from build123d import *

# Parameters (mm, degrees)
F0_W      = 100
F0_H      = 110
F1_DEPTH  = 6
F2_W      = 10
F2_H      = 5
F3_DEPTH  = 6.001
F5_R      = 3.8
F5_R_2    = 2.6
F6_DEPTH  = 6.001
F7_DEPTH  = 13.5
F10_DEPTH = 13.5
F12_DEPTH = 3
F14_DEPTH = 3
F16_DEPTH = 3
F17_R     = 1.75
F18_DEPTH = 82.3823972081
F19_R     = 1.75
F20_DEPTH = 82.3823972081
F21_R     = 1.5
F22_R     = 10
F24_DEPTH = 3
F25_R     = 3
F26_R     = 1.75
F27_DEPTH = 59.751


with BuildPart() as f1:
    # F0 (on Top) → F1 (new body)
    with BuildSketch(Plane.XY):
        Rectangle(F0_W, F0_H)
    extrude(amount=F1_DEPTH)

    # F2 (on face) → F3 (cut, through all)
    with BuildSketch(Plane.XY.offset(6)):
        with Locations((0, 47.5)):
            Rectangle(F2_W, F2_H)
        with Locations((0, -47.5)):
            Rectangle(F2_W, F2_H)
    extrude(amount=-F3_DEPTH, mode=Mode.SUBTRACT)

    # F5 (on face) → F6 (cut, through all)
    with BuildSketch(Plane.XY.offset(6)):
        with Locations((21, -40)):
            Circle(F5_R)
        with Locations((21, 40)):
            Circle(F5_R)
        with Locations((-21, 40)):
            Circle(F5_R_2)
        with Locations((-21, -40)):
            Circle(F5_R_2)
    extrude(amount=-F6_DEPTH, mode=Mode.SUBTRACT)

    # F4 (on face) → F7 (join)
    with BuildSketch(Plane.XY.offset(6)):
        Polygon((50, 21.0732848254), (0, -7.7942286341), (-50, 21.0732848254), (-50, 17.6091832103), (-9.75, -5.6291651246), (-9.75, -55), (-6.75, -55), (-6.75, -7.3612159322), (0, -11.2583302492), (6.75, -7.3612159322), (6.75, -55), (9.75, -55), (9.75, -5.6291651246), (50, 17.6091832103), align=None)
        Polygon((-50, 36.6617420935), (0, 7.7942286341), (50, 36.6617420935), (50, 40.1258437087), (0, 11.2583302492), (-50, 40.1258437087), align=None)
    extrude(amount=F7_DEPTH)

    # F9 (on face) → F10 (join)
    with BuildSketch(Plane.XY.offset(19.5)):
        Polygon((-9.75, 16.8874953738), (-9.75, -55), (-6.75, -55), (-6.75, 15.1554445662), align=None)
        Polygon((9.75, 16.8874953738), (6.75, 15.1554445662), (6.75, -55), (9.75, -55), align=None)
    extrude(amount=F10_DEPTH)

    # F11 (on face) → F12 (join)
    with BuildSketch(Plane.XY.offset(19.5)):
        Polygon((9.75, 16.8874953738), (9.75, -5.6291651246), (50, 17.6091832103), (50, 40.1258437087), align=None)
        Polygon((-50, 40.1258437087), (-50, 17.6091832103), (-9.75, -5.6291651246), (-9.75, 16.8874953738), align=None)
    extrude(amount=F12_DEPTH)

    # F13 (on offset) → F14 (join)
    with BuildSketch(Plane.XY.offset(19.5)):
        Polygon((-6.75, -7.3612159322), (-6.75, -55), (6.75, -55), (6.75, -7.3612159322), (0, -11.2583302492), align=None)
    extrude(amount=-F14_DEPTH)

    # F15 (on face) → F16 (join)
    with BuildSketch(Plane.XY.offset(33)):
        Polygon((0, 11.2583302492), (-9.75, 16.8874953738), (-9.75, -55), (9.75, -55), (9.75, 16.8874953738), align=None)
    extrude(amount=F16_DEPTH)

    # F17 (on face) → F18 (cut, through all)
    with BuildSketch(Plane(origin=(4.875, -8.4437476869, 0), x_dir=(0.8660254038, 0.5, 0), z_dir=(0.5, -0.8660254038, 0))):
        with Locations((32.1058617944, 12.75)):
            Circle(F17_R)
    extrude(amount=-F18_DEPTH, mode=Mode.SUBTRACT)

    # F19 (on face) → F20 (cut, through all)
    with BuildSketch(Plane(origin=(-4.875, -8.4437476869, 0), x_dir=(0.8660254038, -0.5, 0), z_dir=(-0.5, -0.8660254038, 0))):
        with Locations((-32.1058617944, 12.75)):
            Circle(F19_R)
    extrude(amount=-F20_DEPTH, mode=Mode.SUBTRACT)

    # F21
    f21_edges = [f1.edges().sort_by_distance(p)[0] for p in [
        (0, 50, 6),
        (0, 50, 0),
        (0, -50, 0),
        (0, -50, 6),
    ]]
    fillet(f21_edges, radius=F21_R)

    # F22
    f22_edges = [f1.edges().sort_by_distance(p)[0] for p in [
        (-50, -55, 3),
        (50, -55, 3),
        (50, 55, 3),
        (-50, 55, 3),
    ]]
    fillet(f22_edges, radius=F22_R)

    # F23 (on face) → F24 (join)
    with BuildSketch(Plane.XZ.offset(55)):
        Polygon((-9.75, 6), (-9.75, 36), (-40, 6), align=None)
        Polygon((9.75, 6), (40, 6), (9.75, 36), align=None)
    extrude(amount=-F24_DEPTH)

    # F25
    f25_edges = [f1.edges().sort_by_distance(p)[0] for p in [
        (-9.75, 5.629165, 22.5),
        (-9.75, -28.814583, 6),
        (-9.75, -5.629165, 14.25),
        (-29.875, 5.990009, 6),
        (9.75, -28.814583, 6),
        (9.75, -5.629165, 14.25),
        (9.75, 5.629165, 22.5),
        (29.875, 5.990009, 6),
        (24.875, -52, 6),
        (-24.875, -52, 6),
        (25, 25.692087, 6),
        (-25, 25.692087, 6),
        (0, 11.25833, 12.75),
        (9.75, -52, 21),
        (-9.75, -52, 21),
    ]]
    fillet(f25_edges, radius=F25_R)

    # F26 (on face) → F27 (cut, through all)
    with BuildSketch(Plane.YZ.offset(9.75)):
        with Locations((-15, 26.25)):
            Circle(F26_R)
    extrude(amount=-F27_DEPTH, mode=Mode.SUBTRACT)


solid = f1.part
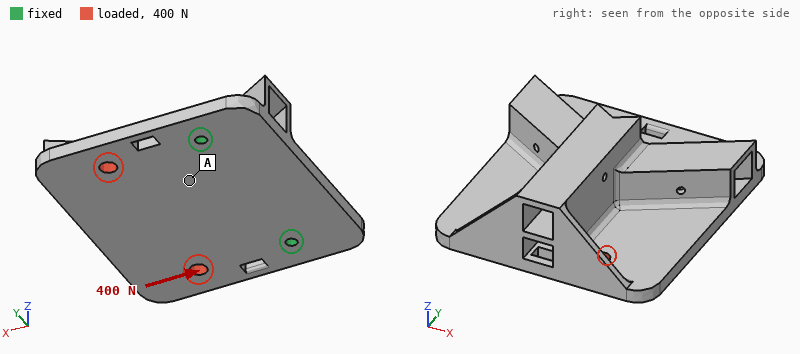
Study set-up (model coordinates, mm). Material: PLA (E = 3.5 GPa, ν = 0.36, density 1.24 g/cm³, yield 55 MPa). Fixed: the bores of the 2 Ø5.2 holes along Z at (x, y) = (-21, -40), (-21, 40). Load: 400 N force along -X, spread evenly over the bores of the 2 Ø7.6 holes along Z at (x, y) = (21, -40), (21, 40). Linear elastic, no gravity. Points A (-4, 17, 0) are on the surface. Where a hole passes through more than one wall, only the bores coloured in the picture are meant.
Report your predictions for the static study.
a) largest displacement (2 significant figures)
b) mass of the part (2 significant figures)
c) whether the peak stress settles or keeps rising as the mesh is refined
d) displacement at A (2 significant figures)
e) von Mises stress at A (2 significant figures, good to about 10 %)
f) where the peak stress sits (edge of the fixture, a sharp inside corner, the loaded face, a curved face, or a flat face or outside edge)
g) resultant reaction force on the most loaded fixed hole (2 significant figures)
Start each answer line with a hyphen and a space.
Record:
- 23 µm
- 120 g
- keeps rising
- 8.6 µm
- 0.29 MPa
- edge of the fixture
- 200 N
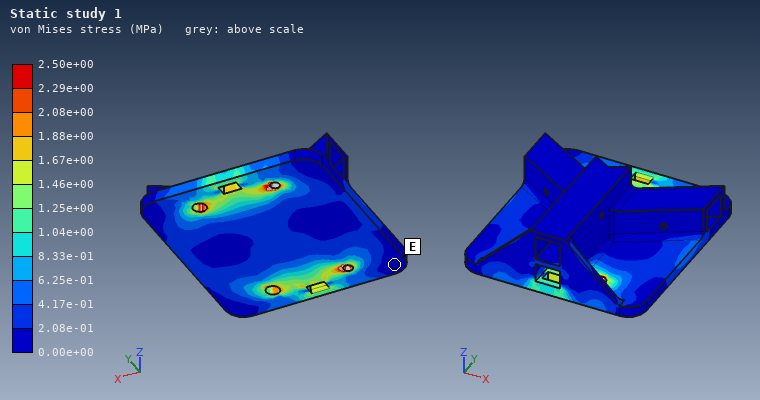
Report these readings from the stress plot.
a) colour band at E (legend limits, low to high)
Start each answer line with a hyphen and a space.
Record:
- 0.00e+00 to 2.08e-01 MPa
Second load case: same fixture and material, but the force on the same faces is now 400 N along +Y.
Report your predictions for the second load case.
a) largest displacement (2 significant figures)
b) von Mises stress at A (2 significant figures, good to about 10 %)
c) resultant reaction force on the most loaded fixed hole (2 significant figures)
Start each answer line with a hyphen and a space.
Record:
- 55 µm
- 1.4 MPa
- 290 N
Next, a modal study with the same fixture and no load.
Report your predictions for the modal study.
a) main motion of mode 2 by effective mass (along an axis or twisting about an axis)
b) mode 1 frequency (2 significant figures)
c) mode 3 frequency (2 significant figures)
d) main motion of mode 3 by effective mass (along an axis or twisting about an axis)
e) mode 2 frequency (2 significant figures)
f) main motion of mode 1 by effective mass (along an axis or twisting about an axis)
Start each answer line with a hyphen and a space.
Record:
- twisting about X
- 310 Hz
- 1400 Hz
- along Z
- 1000 Hz
- along Z
